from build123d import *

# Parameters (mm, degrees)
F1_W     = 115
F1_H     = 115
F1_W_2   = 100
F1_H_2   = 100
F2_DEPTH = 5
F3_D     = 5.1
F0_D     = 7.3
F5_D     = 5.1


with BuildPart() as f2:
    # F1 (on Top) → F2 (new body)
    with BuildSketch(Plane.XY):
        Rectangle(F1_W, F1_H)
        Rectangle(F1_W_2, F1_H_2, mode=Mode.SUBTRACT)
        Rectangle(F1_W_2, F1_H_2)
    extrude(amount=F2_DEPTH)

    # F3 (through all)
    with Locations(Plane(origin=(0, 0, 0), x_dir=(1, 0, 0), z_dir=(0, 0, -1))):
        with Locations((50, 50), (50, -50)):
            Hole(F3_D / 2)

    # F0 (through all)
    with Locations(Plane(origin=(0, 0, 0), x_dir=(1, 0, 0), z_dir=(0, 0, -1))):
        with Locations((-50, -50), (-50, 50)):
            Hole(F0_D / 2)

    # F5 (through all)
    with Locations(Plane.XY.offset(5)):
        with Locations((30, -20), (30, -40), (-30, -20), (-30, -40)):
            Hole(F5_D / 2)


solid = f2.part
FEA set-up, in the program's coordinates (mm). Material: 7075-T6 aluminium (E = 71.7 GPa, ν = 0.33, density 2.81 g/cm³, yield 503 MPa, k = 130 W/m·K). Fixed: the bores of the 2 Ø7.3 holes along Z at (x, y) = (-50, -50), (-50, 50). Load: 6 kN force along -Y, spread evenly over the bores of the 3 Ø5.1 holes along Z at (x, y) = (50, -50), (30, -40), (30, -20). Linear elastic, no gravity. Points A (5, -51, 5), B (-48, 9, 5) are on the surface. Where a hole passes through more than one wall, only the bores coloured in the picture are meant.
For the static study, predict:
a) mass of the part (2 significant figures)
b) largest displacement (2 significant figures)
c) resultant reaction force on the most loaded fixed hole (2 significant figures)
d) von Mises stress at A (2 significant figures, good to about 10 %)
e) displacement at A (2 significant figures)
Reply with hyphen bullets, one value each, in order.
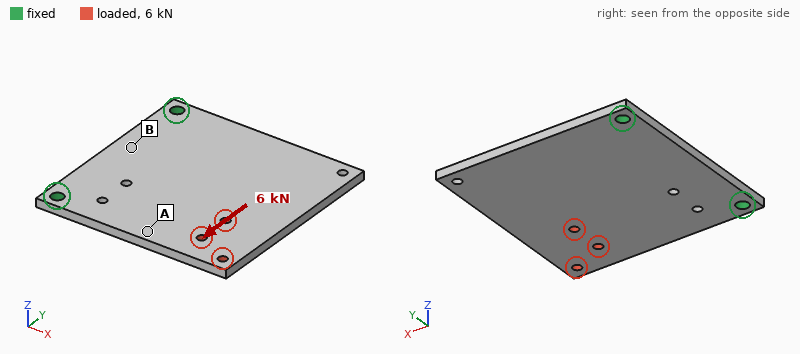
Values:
- 180 g
- 0.11 mm
- 6.0 kN
- 20 MPa
- 0.054 mm
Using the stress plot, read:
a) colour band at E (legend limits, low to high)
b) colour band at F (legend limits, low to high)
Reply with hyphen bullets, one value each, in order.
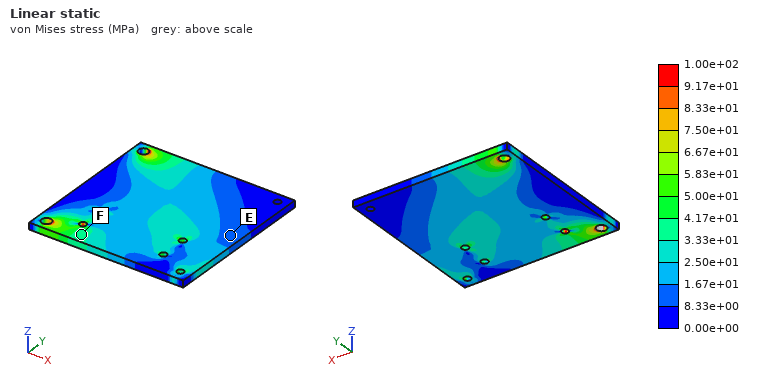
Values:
- 8.33e+00 to 1.67e+01 MPa
- 3.33e+01 to 4.17e+01 MPa
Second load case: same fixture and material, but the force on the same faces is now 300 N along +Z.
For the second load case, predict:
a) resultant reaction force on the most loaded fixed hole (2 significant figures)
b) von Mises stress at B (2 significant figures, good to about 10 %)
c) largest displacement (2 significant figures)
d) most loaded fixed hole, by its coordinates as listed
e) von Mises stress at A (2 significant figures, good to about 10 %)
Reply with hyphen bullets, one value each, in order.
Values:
- 260 N
- 18 MPa
- 1.8 mm
- (-50, -50)
- 32 MPa
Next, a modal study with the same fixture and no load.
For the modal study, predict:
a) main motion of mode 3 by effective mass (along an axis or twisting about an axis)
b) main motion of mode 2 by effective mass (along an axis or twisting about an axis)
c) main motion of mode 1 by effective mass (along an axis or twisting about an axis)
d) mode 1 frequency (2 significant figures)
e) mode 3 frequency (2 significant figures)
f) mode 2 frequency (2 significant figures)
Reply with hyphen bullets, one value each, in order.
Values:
- along Z
- twisting about X
- along Z
- 290 Hz
- 1900 Hz
- 840 Hz
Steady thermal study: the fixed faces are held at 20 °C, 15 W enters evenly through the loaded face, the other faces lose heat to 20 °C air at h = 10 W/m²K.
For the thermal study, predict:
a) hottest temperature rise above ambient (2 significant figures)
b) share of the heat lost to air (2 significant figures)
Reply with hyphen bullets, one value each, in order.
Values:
- 29 K
- 22 %
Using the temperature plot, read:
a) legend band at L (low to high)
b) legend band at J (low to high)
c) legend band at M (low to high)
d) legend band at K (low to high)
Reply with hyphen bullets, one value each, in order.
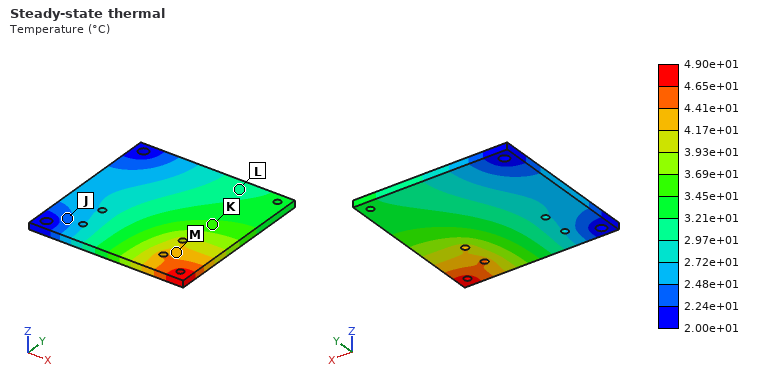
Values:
- 2.97e+01 to 3.21e+01 °C
- 2.24e+01 to 2.48e+01 °C
- 4.17e+01 to 4.41e+01 °C
- 3.45e+01 to 3.69e+01 °C
